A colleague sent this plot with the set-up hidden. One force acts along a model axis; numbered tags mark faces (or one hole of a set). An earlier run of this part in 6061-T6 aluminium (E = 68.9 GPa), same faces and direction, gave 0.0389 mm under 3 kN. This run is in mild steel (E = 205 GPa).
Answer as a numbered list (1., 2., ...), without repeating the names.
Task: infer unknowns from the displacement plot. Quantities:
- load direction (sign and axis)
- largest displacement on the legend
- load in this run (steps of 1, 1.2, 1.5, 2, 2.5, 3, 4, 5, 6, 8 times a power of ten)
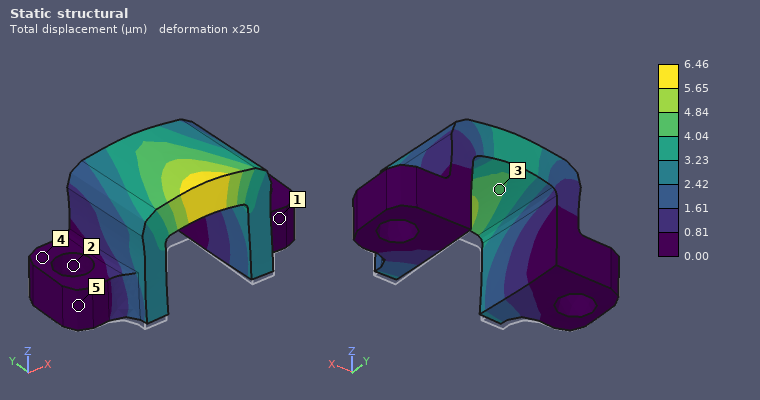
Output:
1. +Z
2. 6.46 µm
3. 1.5 kN
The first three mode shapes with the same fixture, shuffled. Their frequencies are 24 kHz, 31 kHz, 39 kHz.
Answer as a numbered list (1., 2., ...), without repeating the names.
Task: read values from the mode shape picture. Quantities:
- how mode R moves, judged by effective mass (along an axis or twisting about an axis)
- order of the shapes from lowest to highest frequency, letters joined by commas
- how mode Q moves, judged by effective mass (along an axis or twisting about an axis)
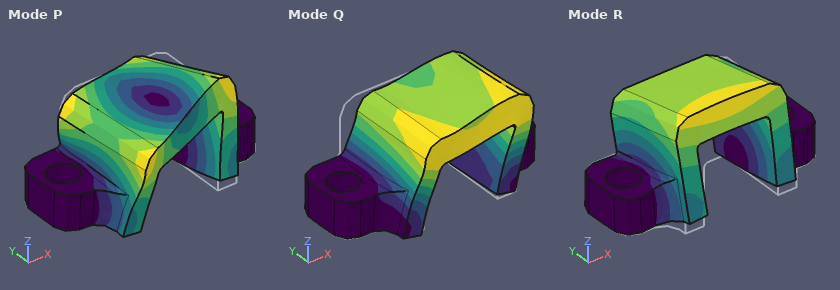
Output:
1. along Y
2. R, Q, P
3. along X
